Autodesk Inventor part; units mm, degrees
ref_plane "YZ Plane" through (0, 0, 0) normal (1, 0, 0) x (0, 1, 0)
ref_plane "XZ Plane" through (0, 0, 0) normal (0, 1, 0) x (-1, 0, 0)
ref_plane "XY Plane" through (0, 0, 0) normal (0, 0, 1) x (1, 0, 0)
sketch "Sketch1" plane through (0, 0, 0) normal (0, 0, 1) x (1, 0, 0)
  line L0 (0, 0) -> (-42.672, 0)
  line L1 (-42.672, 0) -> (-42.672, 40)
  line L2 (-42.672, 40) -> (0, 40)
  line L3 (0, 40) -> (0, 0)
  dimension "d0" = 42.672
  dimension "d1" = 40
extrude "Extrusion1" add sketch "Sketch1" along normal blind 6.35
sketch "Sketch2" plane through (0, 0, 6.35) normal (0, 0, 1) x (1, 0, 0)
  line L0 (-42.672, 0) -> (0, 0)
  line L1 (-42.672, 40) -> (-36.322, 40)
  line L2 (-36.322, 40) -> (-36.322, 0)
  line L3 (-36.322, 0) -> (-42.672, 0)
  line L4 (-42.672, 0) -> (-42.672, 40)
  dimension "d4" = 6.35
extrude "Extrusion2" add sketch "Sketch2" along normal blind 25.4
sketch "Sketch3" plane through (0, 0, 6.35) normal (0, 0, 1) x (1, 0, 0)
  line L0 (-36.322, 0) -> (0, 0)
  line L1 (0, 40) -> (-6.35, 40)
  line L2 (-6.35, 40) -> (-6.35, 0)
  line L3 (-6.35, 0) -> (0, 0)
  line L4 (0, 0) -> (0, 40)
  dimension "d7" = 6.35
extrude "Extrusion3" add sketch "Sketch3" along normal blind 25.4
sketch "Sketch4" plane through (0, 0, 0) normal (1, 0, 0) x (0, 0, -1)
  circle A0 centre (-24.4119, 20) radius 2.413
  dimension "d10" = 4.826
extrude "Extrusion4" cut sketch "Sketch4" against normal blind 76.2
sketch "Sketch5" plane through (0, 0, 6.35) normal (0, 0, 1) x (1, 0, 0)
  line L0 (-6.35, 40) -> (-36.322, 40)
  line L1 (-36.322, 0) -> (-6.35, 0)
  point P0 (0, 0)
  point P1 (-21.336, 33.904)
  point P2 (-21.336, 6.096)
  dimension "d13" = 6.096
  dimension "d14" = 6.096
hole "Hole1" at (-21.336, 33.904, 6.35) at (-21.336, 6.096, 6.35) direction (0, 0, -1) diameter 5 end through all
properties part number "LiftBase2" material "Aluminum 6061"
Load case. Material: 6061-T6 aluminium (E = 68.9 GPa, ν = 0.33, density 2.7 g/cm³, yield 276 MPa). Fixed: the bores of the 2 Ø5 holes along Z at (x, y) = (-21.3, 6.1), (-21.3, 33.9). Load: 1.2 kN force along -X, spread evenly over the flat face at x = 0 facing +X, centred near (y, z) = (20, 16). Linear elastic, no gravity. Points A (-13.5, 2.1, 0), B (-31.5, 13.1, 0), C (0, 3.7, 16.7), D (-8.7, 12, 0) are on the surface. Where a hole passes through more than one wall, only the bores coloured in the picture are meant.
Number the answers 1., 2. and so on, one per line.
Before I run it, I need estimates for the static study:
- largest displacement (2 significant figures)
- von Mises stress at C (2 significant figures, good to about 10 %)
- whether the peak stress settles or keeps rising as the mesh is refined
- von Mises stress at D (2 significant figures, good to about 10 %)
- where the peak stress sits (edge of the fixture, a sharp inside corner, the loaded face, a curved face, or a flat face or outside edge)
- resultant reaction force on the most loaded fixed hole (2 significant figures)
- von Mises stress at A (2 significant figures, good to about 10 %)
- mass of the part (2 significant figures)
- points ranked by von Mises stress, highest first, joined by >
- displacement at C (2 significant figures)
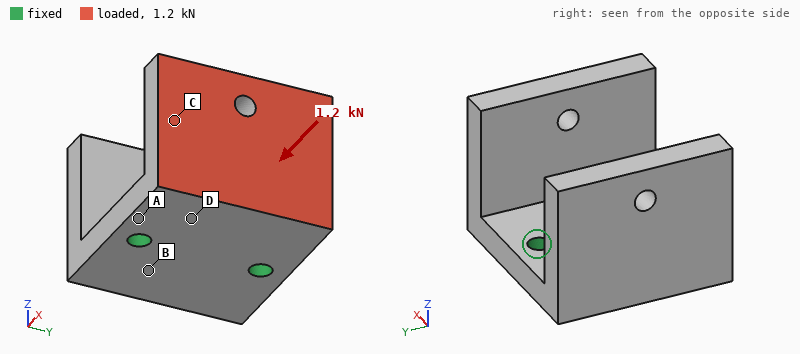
1. 0.18 mm
2. 17 MPa
3. keeps rising
4. 43 MPa
5. edge of the fixture
6. 610 N
7. 56 MPa
8. 63 g
9. A > D > C > B
10. 0.093 mm
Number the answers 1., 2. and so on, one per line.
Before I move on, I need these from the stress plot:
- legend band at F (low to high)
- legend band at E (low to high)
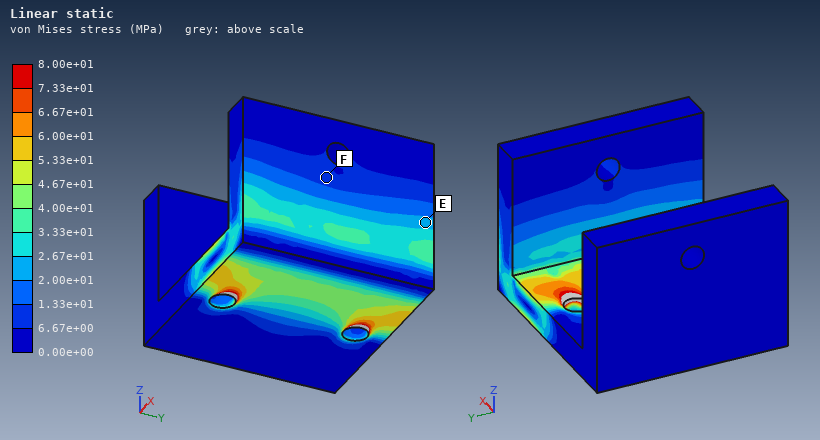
1. 6.67e+00 to 1.33e+01 MPa
2. 2.00e+01 to 2.67e+01 MPa
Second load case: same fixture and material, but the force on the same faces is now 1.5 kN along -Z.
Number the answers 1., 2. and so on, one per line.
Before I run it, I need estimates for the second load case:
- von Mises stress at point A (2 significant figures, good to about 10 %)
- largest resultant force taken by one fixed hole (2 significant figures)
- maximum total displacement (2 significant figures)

1. 85 MPa
2. 750 N
3. 0.20 mm
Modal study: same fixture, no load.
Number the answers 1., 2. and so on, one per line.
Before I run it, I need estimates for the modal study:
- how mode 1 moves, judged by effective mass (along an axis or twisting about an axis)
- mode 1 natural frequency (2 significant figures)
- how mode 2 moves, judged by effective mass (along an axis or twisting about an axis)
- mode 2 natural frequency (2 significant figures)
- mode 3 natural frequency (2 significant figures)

1. along X
2. 3000 Hz
3. along Z
4. 3300 Hz
5. 5800 Hz
